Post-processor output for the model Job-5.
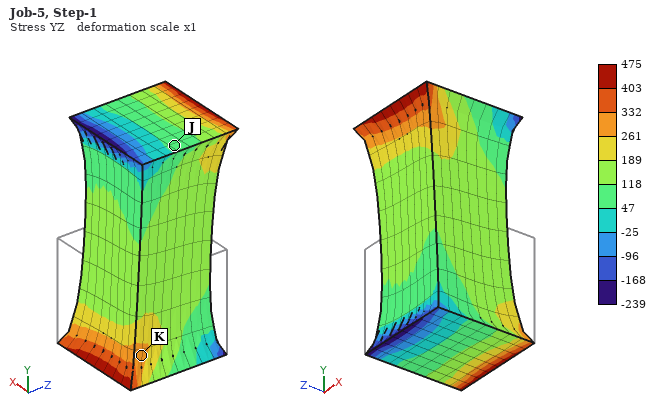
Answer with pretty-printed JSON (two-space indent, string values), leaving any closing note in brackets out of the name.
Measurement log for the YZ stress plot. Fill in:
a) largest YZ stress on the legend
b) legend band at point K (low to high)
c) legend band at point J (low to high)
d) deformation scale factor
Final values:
{
  "largest YZ stress on the legend": "475",
  "legend band at point K": "261 to 332",
  "legend band at point J": "47 to 118",
  "deformation scale factor": "1"
}
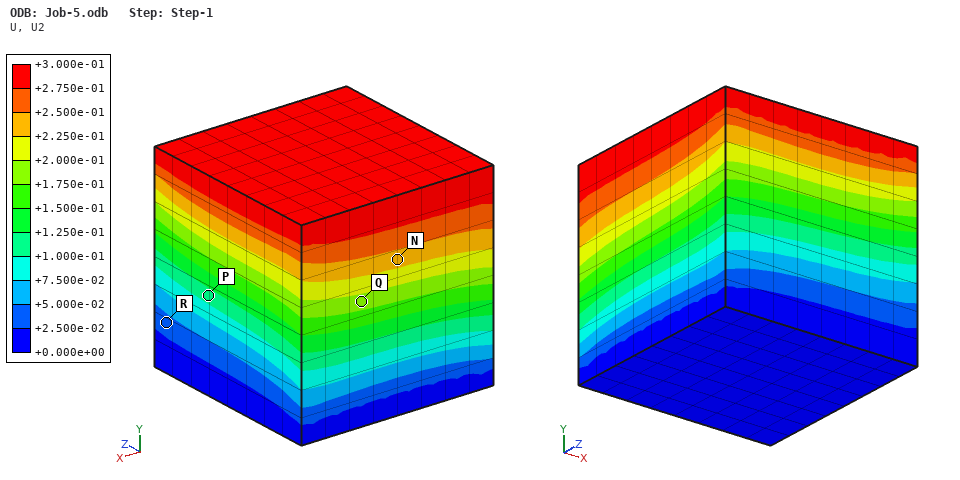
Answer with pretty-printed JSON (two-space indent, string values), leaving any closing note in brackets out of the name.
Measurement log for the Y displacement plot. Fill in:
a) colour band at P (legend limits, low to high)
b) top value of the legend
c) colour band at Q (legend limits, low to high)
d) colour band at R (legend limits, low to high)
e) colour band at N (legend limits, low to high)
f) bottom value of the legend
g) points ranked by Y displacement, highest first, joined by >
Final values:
{
  "colour band at P": "+1.000e-01 to +1.250e-01",
  "top value of the legend": "+3.000e-01",
  "colour band at Q": "+1.750e-01 to +2.000e-01",
  "colour band at R": "+2.500e-02 to +5.000e-02",
  "colour band at N": "+2.250e-01 to +2.500e-01",
  "bottom value of the legend": "+0.000e+00",
  "points ranked by Y displacement, highest first, joined by >": "N > Q > P > R"
}
